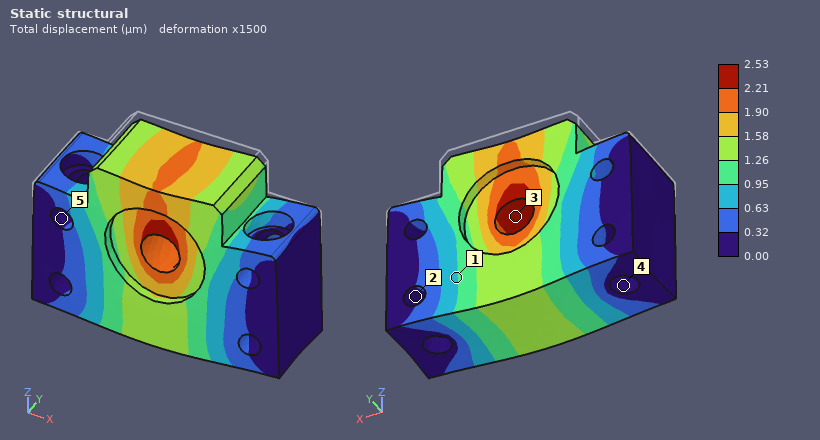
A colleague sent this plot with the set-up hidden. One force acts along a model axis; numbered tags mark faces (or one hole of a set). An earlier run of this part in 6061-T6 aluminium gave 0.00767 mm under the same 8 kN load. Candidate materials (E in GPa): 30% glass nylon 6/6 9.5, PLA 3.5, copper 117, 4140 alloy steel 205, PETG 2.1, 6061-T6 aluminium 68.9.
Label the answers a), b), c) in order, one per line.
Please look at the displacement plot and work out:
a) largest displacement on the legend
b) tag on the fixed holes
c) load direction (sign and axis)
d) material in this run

a) 2.53 µm
b) 4
c) -Z
d) 4140 alloy steel
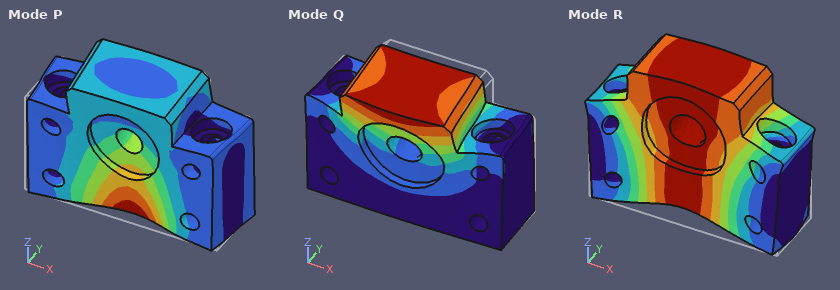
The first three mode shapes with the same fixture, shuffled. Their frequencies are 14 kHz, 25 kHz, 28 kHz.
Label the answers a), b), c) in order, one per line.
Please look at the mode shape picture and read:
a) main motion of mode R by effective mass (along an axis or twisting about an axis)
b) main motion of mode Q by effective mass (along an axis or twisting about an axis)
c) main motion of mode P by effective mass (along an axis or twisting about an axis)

a) along Z
b) along Y
c) along Y
